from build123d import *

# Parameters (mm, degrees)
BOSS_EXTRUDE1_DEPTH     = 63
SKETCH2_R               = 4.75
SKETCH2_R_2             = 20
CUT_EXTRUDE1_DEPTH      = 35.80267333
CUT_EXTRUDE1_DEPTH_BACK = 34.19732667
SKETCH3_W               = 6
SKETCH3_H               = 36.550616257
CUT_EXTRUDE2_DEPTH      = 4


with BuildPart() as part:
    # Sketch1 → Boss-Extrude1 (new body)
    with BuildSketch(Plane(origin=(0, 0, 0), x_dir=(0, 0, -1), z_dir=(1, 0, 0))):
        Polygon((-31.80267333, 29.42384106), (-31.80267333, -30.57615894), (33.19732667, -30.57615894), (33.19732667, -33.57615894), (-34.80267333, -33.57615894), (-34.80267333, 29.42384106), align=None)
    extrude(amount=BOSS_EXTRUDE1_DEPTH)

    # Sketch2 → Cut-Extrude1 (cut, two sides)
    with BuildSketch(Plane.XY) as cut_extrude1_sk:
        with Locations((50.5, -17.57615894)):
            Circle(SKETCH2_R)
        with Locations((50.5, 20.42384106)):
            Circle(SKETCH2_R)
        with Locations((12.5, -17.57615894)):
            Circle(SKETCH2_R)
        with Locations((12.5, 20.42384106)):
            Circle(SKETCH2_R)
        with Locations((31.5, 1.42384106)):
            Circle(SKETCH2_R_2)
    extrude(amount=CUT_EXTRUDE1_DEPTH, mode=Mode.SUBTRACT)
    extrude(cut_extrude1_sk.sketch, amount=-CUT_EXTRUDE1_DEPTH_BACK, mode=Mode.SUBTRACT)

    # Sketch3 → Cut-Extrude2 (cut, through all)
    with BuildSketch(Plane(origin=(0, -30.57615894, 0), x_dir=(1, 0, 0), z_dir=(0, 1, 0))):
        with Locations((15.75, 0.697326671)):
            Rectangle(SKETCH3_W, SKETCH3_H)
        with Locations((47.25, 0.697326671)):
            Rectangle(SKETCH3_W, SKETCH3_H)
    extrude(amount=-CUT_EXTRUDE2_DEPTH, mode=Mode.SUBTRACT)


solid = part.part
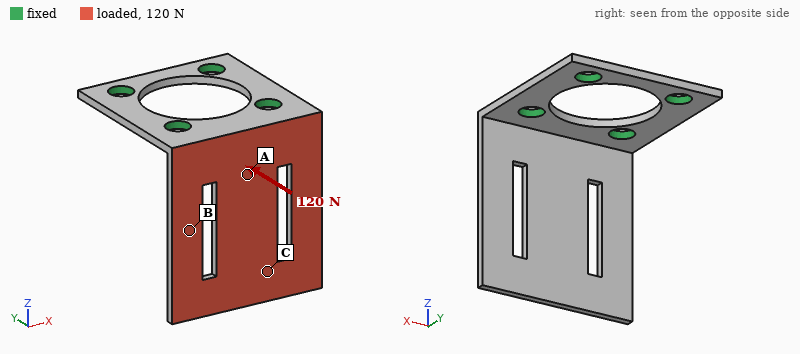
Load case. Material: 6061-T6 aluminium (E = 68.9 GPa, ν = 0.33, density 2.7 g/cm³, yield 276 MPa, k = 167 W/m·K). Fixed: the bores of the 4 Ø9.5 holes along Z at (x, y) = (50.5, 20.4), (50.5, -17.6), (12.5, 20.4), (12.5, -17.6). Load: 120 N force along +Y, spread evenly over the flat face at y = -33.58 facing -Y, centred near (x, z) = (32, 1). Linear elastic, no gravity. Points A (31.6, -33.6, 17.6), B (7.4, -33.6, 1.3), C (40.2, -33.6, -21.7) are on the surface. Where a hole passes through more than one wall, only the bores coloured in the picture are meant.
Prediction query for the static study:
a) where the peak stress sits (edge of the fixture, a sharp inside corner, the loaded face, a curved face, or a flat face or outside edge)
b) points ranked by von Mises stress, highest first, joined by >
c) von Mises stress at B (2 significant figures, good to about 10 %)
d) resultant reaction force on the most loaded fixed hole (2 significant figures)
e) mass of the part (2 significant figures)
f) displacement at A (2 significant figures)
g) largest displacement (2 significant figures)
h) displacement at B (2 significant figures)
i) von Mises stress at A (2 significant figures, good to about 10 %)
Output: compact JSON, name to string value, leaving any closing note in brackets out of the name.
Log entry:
{"where the peak stress sits": "a flat face or outside edge", "points ranked by von Mises stress, highest first, joined by >": "A > B > C", "von Mises stress at B": "15 MPa", "resultant reaction force on the most loaded fixed hole": "65 N", "mass of the part": "49 g", "displacement at A": "0.11 mm", "largest displacement": "0.74 mm", "displacement at B": "0.28 mm", "von Mises stress at A": "25 MPa"}
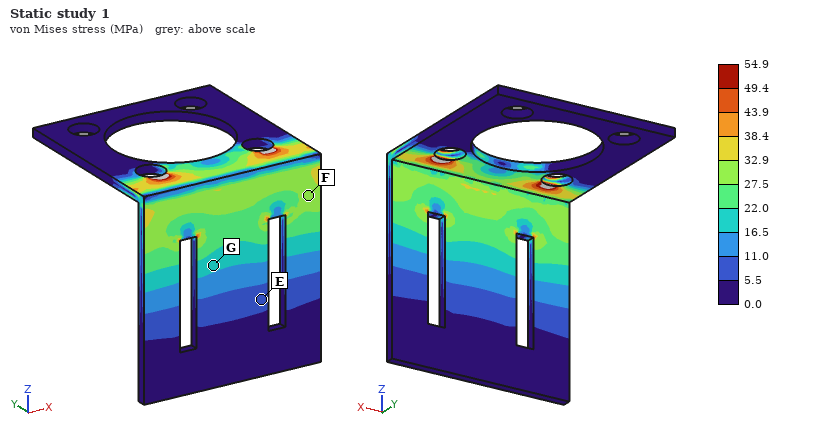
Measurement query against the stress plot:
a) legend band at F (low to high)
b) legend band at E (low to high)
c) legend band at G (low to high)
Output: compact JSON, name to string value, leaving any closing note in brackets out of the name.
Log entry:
{"legend band at F": "27.5 to 32.9 MPa", "legend band at E": "5.5 to 11.0 MPa", "legend band at G": "16.5 to 22.0 MPa"}
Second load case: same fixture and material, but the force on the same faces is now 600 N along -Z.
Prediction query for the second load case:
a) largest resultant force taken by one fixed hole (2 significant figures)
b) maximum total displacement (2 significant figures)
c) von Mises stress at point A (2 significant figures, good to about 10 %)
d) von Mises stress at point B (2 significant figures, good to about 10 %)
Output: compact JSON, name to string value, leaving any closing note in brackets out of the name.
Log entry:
{"largest resultant force taken by one fixed hole": "300 N", "maximum total displacement": "0.49 mm", "von Mises stress at point A": "8.7 MPa", "von Mises stress at point B": "8.0 MPa"}
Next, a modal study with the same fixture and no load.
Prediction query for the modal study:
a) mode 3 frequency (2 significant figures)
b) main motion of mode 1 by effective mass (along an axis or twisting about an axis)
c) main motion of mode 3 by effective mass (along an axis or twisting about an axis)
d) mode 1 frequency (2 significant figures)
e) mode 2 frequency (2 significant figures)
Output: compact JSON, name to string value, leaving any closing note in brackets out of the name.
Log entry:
{"mode 3 frequency": "2100 Hz", "main motion of mode 1 by effective mass": "along Y", "main motion of mode 3 by effective mass": "along X", "mode 1 frequency": "440 Hz", "mode 2 frequency": "1200 Hz"}
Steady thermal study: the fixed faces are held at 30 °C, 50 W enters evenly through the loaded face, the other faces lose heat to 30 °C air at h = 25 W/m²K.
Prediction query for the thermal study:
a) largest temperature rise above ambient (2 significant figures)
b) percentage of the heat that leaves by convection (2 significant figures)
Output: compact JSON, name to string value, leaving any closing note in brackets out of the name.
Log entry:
{"largest temperature rise above ambient": "68 K", "percentage of the heat that leaves by convection": "13 %"}
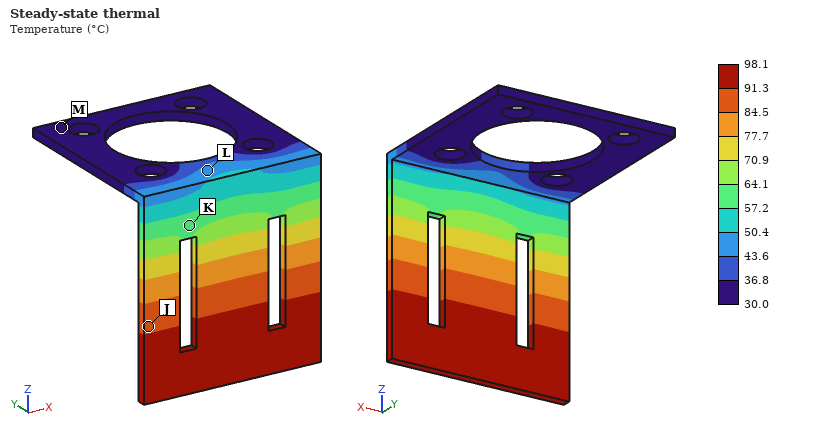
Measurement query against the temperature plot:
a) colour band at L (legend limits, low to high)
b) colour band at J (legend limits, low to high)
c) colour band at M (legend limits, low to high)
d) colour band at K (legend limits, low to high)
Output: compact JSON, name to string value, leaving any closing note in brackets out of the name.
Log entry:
{"colour band at L": "43.6 to 50.4 °C", "colour band at J": "84.5 to 91.3 °C", "colour band at M": "30.0 to 36.8 °C", "colour band at K": "57.2 to 64.1 °C"}
